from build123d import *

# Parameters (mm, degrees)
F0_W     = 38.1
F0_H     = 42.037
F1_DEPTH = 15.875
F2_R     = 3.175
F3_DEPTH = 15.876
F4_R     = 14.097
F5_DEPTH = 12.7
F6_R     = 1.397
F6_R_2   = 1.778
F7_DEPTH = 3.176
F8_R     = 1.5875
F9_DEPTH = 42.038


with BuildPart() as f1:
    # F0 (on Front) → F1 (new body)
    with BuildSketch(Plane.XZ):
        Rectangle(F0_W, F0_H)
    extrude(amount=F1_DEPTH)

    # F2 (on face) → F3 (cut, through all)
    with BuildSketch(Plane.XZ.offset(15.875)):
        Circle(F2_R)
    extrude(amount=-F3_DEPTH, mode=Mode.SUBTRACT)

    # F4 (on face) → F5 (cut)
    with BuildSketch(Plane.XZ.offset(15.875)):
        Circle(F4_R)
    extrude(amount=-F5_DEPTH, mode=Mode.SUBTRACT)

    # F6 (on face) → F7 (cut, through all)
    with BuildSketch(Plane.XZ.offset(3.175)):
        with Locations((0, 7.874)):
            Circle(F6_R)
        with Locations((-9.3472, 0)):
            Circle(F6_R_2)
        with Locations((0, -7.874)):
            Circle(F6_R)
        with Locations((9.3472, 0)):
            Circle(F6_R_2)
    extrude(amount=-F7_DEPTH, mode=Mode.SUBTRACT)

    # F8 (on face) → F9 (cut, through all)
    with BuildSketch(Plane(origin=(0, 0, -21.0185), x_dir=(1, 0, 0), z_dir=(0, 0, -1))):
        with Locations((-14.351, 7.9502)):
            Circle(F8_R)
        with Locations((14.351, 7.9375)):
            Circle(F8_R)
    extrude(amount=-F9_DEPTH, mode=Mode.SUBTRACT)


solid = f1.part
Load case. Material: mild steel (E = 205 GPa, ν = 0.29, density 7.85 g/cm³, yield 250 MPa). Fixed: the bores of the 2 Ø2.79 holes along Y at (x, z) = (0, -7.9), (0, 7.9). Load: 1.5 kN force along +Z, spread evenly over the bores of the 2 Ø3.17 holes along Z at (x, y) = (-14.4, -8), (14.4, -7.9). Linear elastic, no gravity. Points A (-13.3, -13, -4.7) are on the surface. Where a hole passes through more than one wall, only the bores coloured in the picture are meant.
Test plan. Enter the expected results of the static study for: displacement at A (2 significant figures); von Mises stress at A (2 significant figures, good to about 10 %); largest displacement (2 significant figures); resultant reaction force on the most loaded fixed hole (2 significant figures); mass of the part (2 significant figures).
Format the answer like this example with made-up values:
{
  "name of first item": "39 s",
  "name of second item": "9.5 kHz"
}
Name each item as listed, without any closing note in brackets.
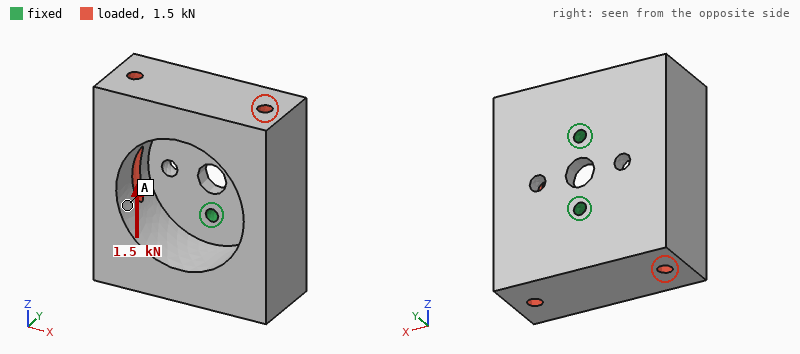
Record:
{
  "displacement at A": "5.7 µm",
  "von Mises stress at A": "8.2 MPa",
  "largest displacement": "9.6 µm",
  "resultant reaction force on the most loaded fixed hole": "870 N",
  "mass of the part": "130 g"
}
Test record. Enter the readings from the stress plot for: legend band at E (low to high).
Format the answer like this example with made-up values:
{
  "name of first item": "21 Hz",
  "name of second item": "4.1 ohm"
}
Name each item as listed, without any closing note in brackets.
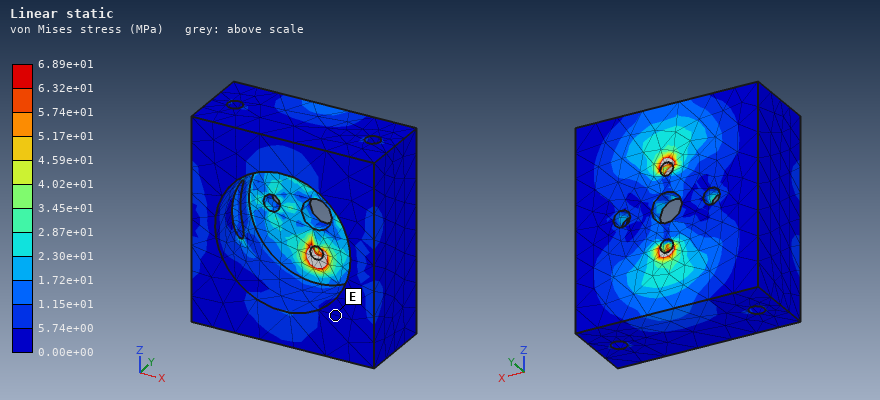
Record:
{
  "legend band at E": "0.00e+00 to 5.74e+00 MPa"
}
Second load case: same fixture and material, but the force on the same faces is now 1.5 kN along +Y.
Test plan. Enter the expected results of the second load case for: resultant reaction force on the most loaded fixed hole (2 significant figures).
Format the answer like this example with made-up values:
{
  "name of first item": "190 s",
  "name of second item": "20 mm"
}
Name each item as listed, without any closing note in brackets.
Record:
{
  "resultant reaction force on the most loaded fixed hole": "760 N"
}
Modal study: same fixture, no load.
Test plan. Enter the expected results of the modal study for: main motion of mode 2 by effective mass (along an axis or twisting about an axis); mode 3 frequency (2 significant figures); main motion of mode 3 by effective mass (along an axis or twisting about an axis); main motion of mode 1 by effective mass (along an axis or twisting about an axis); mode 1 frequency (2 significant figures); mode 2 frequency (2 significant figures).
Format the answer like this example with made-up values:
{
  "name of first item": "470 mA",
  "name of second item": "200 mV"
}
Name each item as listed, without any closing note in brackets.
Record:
{
  "main motion of mode 2 by effective mass": "along Z",
  "mode 3 frequency": "8000 Hz",
  "main motion of mode 3 by effective mass": "twisting about Y",
  "main motion of mode 1 by effective mass": "along X",
  "mode 1 frequency": "2600 Hz",
  "mode 2 frequency": "5200 Hz"
}
